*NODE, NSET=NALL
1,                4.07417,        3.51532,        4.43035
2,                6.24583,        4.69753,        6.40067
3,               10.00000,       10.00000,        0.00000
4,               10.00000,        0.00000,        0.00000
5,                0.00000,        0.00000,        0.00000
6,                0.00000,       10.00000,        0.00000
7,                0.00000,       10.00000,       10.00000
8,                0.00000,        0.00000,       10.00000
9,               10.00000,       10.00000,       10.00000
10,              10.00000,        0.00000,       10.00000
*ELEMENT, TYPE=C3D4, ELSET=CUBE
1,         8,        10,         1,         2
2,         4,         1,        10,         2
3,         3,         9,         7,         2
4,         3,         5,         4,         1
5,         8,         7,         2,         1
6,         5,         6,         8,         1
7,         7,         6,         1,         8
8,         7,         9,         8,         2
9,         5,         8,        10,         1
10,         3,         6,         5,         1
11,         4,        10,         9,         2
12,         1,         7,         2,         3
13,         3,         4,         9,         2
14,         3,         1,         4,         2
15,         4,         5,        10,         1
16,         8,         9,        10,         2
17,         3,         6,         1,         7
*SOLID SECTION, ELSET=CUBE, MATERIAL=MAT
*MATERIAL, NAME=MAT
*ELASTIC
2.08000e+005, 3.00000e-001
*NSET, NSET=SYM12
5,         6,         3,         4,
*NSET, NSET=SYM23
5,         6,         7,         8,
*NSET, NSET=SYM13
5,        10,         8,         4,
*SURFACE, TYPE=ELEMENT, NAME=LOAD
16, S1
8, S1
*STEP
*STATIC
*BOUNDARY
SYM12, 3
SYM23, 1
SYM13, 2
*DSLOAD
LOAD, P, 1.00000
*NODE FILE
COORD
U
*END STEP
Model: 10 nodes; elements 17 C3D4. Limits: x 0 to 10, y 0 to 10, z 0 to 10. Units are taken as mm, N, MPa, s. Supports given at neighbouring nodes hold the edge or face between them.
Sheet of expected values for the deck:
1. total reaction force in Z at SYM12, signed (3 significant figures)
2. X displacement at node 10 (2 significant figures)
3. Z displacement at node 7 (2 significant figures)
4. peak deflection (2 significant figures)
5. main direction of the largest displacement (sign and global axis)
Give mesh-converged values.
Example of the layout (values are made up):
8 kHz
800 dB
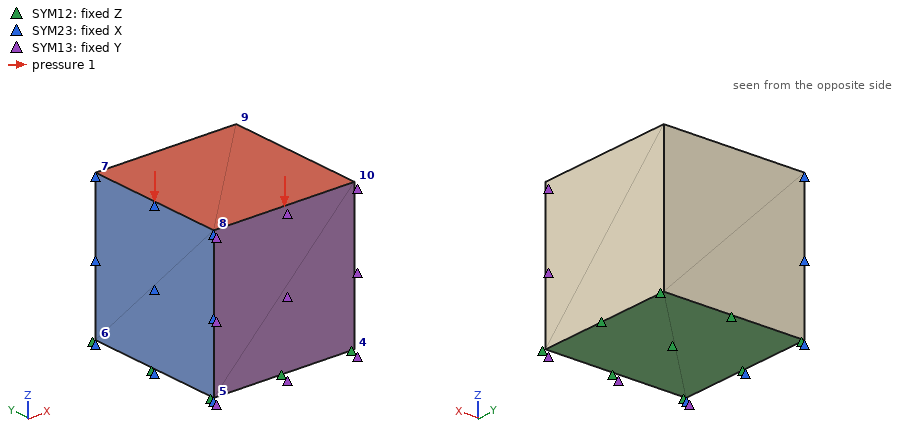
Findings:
100 N
1.4e-05 mm
-4.8e-05 mm
5.2e-05 mm
-Z
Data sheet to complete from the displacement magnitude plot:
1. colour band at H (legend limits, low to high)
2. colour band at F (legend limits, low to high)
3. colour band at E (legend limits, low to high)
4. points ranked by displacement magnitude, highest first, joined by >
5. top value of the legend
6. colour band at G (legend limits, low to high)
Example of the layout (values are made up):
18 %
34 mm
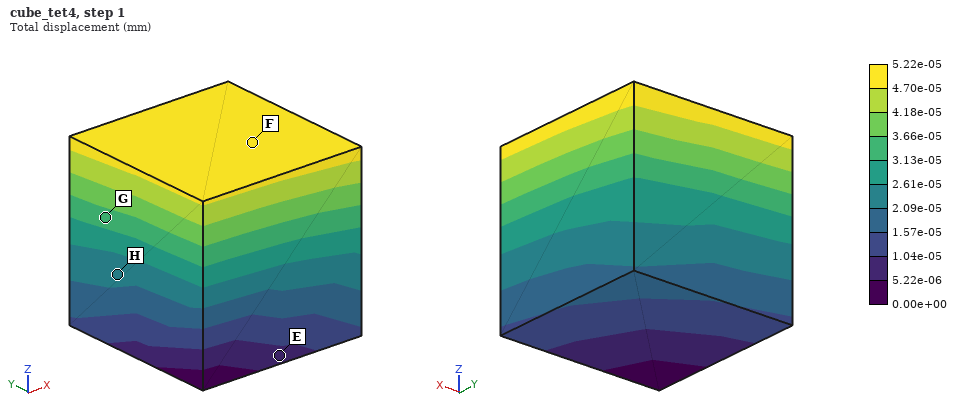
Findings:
2.09e-05 to 2.61e-05 mm
4.70e-05 to 5.22e-05 mm
5.22e-06 to 1.04e-05 mm
F > G > H > E
5.22e-05 mm
3.13e-05 to 3.66e-05 mm
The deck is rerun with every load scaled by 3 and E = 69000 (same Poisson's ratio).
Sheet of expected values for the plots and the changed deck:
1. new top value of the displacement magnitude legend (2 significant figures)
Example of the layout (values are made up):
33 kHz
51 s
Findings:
4.7e-04 mm
